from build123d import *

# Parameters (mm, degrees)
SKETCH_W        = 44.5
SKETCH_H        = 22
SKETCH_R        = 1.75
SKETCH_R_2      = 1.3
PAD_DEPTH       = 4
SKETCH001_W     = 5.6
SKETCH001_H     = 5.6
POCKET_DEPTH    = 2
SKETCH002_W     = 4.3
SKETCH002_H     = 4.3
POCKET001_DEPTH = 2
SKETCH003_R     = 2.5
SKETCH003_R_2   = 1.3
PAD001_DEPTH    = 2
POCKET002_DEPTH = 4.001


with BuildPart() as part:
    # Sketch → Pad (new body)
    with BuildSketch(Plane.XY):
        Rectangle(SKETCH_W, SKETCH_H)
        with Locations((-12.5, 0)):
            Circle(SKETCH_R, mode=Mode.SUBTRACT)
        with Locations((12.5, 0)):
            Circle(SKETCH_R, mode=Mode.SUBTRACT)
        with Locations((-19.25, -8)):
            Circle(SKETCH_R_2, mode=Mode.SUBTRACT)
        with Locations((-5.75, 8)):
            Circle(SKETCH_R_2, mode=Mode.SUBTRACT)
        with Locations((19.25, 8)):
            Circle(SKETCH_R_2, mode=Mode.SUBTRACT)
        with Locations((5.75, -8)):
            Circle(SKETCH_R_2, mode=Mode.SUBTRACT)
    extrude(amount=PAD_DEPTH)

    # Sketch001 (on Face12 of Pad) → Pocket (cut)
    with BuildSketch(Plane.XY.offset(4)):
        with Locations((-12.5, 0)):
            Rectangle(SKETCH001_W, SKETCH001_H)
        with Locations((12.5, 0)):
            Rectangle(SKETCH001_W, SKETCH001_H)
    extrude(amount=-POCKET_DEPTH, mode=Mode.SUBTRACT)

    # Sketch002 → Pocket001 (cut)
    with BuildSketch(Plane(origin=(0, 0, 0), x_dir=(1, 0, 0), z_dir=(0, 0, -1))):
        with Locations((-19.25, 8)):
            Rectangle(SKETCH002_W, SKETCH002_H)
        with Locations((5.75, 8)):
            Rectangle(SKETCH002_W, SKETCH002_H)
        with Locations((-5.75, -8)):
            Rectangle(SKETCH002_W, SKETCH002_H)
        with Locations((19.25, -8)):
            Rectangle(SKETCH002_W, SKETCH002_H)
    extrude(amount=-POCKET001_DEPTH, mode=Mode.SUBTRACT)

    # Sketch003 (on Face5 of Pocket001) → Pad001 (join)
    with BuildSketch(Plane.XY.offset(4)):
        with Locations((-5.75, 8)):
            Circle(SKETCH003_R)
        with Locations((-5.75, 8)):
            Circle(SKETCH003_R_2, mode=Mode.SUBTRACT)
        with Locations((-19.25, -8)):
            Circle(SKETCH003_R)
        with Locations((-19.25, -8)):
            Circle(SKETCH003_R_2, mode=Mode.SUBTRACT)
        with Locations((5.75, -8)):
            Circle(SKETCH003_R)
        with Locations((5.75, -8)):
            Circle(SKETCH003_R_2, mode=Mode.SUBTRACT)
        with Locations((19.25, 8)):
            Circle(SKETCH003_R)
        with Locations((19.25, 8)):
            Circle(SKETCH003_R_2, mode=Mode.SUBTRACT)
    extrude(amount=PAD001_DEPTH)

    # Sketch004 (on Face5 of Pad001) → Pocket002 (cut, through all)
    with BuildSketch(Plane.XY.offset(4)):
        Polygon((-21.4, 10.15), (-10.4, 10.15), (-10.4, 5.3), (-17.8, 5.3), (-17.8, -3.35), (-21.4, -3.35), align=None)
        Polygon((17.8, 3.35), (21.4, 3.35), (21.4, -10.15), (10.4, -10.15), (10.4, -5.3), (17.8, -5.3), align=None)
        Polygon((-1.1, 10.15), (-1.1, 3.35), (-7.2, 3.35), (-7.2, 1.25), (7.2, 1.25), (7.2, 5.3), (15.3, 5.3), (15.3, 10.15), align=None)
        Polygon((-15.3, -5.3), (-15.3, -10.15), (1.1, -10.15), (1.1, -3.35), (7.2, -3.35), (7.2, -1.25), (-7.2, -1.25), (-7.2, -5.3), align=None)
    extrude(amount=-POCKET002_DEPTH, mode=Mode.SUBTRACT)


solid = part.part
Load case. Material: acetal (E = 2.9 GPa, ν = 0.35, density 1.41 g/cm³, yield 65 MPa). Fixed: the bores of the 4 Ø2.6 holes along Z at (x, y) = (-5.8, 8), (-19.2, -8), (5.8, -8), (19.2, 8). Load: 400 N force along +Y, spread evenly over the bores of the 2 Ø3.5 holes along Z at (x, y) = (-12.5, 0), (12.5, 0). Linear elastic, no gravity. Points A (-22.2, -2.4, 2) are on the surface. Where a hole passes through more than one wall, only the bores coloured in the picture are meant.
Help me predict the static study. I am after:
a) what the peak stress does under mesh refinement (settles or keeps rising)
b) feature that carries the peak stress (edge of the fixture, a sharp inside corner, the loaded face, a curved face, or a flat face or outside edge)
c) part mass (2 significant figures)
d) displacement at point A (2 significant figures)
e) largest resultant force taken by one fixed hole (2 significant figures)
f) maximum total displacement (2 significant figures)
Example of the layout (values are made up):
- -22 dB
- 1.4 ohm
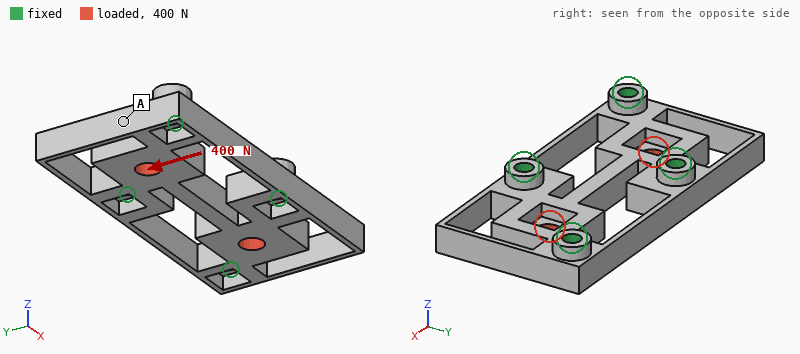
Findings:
- keeps rising
- edge of the fixture
- 2.8 g
- 30 µm
- 110 N
- 94 µm
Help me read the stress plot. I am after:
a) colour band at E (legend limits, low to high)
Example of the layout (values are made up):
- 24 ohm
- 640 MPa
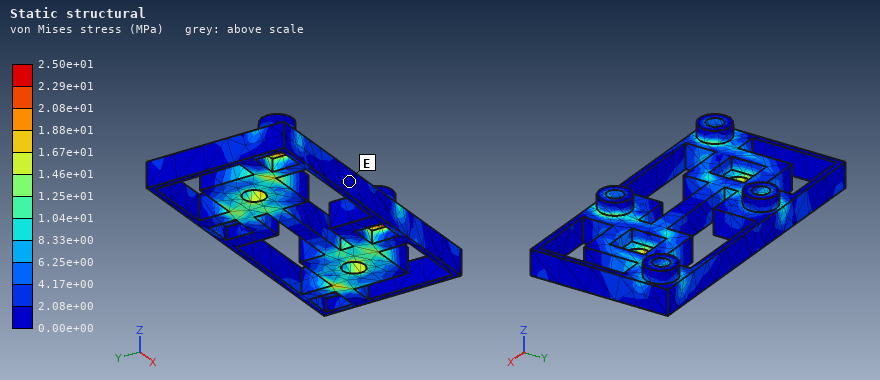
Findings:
- 0.00e+00 to 2.08e+00 MPa
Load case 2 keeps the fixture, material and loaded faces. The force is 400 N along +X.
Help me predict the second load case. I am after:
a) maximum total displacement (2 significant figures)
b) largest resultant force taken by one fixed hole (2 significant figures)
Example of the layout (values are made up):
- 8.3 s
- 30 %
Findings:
- 0.11 mm
- 100 N
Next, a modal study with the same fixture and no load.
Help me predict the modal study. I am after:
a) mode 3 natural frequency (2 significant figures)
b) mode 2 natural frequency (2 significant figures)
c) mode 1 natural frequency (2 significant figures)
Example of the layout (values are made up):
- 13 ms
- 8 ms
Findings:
- 4200 Hz
- 3900 Hz
- 3900 Hz
